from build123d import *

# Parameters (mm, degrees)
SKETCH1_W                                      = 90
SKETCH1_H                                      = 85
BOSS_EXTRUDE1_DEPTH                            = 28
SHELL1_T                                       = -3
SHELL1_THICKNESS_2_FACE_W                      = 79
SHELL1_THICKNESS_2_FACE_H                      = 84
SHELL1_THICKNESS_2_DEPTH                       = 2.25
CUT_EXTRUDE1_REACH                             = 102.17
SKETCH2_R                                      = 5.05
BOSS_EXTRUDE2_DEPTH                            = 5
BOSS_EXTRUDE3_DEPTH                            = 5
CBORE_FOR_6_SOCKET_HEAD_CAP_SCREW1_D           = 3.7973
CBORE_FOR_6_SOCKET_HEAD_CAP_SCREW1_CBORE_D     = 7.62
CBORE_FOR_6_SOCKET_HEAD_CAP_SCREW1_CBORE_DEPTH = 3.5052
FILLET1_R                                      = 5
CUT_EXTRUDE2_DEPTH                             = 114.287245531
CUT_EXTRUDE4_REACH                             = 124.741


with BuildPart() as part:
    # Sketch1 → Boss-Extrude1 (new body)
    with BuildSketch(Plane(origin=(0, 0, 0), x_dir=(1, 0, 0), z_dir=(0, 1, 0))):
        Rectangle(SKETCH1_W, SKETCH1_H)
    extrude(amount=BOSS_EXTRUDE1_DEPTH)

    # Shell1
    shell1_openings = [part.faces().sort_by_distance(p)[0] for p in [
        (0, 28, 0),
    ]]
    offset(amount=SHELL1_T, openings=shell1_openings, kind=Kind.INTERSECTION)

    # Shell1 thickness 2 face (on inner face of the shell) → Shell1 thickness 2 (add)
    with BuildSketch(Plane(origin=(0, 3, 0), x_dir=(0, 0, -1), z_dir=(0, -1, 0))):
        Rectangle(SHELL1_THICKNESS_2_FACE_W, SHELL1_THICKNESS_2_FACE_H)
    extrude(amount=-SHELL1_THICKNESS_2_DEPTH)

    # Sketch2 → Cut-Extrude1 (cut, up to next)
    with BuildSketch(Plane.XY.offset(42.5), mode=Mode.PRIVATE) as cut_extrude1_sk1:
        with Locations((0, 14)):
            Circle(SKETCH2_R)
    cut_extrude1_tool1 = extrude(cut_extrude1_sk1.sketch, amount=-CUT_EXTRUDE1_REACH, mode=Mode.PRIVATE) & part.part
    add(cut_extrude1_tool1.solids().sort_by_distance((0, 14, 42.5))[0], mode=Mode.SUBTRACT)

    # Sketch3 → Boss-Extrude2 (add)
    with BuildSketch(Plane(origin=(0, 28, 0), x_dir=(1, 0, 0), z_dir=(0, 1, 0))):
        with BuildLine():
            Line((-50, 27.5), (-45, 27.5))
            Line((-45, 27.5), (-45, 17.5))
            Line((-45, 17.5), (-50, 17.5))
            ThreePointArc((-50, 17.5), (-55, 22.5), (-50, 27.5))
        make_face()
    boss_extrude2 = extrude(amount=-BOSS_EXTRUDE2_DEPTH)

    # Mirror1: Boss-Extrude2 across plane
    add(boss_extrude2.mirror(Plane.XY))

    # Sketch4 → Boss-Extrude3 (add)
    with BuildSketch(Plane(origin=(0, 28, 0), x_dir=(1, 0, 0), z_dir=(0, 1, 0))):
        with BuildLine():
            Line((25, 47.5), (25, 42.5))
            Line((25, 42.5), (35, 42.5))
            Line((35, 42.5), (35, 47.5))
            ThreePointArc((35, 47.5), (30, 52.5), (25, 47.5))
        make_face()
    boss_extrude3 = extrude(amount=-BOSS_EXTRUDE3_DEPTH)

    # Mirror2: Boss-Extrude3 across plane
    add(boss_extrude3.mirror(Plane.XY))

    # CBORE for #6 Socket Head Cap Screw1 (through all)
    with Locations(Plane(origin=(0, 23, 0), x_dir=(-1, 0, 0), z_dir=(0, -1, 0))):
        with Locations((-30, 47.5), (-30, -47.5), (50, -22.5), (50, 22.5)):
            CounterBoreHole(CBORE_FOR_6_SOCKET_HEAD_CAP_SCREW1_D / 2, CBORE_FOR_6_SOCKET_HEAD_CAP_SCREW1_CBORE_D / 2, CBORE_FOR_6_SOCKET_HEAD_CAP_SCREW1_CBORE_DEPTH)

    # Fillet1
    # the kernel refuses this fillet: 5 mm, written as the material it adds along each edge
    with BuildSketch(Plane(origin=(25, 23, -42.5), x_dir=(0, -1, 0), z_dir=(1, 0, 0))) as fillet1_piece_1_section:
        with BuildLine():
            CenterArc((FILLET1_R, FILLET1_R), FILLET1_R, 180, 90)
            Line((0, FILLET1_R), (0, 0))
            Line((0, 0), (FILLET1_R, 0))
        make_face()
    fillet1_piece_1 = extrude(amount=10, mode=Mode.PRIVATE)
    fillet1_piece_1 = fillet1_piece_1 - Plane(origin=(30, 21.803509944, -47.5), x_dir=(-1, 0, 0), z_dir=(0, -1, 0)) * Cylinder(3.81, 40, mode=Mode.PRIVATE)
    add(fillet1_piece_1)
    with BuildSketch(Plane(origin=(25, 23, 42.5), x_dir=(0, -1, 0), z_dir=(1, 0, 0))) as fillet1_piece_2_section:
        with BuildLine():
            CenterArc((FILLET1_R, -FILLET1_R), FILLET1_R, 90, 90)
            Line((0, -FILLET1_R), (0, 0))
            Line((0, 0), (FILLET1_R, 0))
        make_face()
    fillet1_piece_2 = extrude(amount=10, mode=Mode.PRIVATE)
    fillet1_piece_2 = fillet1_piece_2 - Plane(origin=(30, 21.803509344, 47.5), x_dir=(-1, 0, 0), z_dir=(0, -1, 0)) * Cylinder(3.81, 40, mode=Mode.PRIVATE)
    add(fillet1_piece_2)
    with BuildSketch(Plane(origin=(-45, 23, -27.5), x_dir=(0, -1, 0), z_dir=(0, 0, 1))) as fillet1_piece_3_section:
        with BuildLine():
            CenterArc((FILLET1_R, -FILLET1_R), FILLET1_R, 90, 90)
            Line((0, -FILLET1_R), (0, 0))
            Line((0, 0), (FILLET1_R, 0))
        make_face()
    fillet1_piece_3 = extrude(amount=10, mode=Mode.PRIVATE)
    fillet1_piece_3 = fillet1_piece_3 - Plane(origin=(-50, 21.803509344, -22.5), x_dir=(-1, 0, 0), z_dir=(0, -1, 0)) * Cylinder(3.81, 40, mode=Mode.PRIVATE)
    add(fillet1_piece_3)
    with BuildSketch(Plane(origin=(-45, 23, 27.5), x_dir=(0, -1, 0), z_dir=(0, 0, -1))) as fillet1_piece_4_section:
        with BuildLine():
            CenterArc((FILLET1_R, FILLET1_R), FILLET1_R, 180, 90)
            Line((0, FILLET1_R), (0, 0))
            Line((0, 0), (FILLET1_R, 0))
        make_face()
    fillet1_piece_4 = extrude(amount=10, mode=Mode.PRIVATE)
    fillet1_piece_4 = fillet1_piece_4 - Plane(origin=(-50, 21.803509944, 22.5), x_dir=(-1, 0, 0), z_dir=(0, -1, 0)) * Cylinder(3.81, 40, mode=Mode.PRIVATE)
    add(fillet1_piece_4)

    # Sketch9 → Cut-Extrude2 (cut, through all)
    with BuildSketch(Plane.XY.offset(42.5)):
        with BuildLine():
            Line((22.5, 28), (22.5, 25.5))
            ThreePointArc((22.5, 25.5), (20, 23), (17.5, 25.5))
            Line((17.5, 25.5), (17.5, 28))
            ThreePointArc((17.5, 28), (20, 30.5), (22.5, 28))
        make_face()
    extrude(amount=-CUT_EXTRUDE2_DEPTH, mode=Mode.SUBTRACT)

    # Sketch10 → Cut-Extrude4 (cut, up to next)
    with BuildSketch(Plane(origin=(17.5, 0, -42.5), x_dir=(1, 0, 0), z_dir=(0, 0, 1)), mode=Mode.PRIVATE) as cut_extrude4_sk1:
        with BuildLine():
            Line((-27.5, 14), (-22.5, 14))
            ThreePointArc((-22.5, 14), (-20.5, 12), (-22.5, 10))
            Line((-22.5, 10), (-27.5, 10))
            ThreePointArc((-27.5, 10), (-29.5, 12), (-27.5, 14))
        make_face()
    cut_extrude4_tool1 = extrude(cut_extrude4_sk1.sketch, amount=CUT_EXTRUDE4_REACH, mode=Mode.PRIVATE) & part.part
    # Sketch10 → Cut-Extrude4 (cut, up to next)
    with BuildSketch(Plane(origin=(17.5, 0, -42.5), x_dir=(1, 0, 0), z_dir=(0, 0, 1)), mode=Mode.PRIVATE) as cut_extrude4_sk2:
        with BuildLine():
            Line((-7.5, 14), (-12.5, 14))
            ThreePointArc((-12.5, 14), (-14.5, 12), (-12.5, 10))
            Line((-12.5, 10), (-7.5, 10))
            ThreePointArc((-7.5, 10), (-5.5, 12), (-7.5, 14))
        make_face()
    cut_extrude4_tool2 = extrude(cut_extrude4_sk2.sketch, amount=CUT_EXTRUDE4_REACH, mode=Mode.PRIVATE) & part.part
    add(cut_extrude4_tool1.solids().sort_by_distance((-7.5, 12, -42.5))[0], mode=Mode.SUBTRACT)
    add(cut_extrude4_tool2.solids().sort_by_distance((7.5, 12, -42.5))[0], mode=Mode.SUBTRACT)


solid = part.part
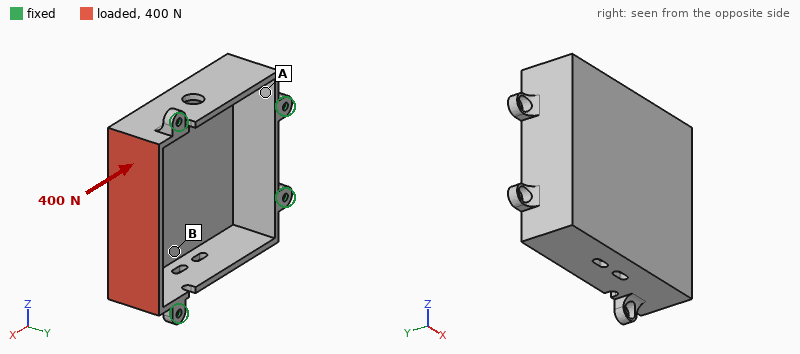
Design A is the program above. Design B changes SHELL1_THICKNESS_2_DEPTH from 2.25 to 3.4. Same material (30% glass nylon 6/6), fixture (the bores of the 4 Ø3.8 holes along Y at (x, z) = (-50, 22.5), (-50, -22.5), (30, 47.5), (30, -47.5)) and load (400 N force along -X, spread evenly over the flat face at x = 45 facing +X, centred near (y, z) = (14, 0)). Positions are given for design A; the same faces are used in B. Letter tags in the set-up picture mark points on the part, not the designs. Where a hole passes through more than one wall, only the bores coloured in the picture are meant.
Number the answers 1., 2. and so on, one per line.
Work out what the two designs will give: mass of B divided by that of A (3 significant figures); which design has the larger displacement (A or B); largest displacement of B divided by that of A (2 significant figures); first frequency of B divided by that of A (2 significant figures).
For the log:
1. 1.12
2. A
3. 0.82
4. 0.97
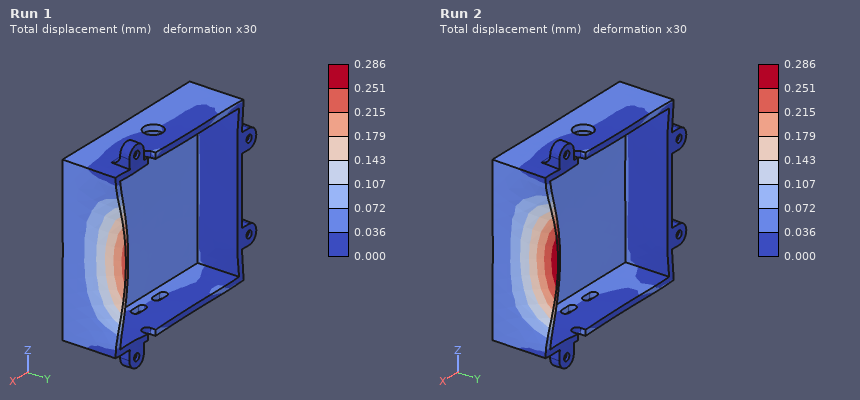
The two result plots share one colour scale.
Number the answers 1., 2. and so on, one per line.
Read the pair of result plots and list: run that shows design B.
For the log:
1. Run 1
